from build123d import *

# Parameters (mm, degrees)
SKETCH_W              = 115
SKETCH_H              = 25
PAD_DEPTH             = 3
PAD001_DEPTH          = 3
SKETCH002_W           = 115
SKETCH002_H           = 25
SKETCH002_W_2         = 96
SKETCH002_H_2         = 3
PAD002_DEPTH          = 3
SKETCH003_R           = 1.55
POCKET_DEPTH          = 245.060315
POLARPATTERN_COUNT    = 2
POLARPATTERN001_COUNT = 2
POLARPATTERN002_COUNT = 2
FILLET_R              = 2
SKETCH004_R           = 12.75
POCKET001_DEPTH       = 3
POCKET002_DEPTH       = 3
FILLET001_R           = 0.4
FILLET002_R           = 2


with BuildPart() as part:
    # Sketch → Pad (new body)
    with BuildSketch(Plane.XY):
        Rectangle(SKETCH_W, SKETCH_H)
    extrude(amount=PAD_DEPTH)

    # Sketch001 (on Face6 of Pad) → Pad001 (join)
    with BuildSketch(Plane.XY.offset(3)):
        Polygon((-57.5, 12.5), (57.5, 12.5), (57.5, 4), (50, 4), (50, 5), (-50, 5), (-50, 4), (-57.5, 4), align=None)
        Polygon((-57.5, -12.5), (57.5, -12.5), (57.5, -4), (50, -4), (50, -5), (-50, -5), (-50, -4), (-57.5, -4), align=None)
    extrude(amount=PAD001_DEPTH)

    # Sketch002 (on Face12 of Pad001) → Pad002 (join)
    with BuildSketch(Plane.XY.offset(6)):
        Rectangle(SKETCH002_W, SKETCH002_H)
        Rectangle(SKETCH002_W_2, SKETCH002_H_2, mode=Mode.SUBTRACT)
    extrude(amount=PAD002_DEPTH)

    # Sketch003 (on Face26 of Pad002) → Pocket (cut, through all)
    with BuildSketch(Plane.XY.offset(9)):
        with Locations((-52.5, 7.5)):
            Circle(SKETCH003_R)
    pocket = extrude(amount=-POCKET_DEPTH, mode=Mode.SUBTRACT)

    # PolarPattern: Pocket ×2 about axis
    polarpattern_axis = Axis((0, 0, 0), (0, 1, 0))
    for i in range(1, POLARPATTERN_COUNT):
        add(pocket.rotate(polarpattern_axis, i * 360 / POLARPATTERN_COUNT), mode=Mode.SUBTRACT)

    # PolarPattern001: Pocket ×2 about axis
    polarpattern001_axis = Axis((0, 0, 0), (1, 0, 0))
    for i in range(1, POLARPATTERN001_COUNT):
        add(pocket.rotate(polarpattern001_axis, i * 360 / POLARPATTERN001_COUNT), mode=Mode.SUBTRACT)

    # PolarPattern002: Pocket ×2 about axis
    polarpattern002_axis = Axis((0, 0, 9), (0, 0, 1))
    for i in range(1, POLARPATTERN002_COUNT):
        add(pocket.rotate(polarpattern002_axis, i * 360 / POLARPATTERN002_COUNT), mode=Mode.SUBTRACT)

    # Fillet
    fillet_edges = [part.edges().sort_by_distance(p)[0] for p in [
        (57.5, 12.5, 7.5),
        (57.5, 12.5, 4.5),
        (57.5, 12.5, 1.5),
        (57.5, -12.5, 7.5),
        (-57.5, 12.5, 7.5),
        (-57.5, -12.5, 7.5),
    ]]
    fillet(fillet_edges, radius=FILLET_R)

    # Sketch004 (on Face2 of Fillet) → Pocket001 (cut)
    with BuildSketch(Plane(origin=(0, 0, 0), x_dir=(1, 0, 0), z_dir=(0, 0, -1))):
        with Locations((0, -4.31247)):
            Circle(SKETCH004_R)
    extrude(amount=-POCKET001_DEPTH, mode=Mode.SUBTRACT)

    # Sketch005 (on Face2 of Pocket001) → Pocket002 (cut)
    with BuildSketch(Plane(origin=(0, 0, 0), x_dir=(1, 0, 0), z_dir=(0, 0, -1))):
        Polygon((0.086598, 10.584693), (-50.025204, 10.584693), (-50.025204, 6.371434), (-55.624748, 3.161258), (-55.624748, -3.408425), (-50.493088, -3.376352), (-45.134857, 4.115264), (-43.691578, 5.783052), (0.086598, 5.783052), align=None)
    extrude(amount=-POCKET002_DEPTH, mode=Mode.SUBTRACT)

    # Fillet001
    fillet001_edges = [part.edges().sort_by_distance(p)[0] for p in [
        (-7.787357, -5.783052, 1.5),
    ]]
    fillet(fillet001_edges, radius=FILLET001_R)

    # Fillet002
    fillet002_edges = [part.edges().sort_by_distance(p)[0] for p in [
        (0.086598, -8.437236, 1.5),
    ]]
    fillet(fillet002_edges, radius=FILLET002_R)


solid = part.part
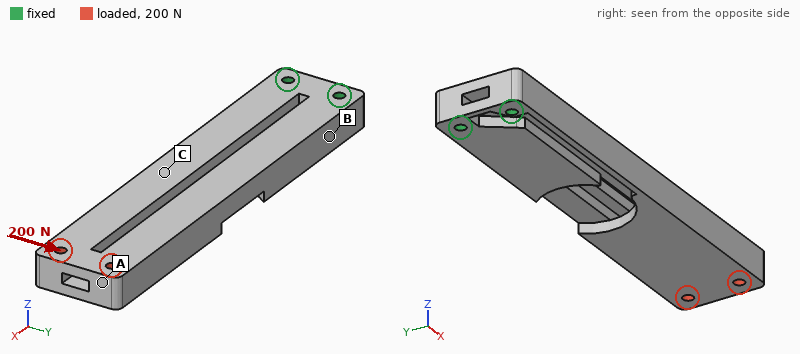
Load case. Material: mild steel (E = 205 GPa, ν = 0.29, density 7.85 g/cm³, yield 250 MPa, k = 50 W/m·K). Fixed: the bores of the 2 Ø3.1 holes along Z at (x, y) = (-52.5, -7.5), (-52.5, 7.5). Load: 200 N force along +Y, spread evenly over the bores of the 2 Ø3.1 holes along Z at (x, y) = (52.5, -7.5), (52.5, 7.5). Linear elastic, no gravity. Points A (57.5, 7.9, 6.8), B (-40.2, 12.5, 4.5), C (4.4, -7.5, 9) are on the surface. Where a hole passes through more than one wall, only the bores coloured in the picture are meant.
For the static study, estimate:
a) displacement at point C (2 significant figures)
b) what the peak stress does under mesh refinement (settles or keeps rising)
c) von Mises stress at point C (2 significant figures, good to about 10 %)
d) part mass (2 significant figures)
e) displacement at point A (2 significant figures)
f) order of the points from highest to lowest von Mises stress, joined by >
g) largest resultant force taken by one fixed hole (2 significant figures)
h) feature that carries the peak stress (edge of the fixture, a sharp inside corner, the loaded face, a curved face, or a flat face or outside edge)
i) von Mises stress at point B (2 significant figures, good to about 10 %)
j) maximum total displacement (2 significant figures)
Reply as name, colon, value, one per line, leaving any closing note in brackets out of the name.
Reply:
displacement at point C: 25 µm
what the peak stress does under mesh refinement: keeps rising
von Mises stress at point C: 11 MPa
part mass: 150 g
displacement at point A: 59 µm
order of the points from highest to lowest von Mises stress, joined by >: B > C > A
largest resultant force taken by one fixed hole: 1.2 kN
feature that carries the peak stress: a sharp inside corner
von Mises stress at point B: 21 MPa
maximum total displacement: 61 µm
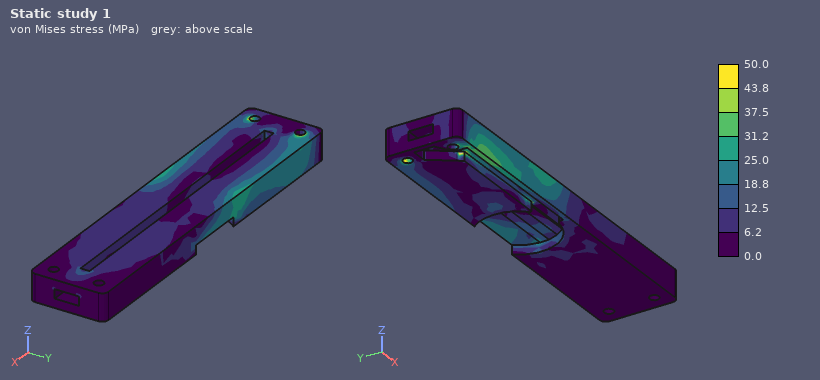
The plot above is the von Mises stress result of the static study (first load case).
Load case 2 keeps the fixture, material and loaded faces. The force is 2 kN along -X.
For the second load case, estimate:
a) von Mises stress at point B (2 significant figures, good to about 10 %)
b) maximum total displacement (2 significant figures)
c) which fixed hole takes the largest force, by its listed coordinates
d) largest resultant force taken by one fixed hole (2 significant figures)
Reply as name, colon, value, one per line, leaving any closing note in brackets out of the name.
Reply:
von Mises stress at point B: 11 MPa
maximum total displacement: 69 µm
which fixed hole takes the largest force, by its listed coordinates: (-52.5, 7.5)
largest resultant force taken by one fixed hole: 1.1 kN
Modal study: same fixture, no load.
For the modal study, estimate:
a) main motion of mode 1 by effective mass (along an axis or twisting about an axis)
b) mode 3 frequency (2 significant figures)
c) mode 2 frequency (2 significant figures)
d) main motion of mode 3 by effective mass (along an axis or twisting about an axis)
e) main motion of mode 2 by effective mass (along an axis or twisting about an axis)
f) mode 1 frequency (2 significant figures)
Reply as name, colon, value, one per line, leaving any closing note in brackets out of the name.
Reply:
main motion of mode 1 by effective mass: along Z
mode 3 frequency: 2600 Hz
mode 2 frequency: 1400 Hz
main motion of mode 3 by effective mass: twisting about X
main motion of mode 2 by effective mass: along Y
mode 1 frequency: 520 Hz
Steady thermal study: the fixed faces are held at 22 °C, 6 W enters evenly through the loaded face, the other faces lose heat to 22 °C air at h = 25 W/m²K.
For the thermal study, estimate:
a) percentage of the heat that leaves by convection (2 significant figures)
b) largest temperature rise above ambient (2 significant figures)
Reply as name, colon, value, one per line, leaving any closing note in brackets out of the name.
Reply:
percentage of the heat that leaves by convection: 71 %
largest temperature rise above ambient: 38 K
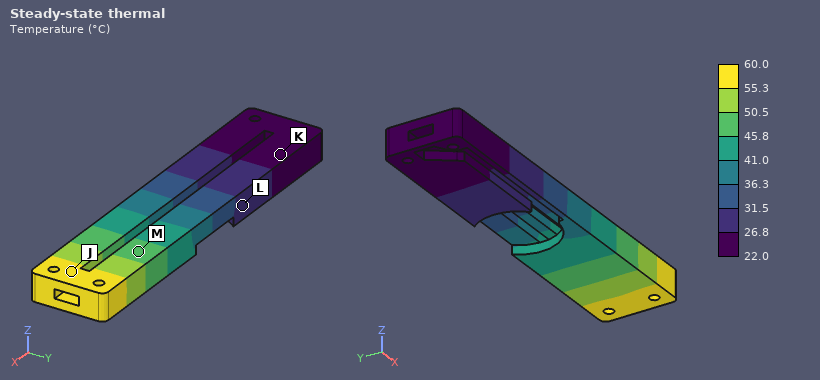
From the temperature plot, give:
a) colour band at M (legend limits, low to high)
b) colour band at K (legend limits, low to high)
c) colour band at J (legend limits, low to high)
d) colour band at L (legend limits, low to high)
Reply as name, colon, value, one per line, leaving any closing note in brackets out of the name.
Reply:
colour band at M: 45.8 to 50.5 °C
colour band at K: 22.0 to 26.8 °C
colour band at J: 55.3 to 60.0 °C
colour band at L: 26.8 to 31.5 °C
